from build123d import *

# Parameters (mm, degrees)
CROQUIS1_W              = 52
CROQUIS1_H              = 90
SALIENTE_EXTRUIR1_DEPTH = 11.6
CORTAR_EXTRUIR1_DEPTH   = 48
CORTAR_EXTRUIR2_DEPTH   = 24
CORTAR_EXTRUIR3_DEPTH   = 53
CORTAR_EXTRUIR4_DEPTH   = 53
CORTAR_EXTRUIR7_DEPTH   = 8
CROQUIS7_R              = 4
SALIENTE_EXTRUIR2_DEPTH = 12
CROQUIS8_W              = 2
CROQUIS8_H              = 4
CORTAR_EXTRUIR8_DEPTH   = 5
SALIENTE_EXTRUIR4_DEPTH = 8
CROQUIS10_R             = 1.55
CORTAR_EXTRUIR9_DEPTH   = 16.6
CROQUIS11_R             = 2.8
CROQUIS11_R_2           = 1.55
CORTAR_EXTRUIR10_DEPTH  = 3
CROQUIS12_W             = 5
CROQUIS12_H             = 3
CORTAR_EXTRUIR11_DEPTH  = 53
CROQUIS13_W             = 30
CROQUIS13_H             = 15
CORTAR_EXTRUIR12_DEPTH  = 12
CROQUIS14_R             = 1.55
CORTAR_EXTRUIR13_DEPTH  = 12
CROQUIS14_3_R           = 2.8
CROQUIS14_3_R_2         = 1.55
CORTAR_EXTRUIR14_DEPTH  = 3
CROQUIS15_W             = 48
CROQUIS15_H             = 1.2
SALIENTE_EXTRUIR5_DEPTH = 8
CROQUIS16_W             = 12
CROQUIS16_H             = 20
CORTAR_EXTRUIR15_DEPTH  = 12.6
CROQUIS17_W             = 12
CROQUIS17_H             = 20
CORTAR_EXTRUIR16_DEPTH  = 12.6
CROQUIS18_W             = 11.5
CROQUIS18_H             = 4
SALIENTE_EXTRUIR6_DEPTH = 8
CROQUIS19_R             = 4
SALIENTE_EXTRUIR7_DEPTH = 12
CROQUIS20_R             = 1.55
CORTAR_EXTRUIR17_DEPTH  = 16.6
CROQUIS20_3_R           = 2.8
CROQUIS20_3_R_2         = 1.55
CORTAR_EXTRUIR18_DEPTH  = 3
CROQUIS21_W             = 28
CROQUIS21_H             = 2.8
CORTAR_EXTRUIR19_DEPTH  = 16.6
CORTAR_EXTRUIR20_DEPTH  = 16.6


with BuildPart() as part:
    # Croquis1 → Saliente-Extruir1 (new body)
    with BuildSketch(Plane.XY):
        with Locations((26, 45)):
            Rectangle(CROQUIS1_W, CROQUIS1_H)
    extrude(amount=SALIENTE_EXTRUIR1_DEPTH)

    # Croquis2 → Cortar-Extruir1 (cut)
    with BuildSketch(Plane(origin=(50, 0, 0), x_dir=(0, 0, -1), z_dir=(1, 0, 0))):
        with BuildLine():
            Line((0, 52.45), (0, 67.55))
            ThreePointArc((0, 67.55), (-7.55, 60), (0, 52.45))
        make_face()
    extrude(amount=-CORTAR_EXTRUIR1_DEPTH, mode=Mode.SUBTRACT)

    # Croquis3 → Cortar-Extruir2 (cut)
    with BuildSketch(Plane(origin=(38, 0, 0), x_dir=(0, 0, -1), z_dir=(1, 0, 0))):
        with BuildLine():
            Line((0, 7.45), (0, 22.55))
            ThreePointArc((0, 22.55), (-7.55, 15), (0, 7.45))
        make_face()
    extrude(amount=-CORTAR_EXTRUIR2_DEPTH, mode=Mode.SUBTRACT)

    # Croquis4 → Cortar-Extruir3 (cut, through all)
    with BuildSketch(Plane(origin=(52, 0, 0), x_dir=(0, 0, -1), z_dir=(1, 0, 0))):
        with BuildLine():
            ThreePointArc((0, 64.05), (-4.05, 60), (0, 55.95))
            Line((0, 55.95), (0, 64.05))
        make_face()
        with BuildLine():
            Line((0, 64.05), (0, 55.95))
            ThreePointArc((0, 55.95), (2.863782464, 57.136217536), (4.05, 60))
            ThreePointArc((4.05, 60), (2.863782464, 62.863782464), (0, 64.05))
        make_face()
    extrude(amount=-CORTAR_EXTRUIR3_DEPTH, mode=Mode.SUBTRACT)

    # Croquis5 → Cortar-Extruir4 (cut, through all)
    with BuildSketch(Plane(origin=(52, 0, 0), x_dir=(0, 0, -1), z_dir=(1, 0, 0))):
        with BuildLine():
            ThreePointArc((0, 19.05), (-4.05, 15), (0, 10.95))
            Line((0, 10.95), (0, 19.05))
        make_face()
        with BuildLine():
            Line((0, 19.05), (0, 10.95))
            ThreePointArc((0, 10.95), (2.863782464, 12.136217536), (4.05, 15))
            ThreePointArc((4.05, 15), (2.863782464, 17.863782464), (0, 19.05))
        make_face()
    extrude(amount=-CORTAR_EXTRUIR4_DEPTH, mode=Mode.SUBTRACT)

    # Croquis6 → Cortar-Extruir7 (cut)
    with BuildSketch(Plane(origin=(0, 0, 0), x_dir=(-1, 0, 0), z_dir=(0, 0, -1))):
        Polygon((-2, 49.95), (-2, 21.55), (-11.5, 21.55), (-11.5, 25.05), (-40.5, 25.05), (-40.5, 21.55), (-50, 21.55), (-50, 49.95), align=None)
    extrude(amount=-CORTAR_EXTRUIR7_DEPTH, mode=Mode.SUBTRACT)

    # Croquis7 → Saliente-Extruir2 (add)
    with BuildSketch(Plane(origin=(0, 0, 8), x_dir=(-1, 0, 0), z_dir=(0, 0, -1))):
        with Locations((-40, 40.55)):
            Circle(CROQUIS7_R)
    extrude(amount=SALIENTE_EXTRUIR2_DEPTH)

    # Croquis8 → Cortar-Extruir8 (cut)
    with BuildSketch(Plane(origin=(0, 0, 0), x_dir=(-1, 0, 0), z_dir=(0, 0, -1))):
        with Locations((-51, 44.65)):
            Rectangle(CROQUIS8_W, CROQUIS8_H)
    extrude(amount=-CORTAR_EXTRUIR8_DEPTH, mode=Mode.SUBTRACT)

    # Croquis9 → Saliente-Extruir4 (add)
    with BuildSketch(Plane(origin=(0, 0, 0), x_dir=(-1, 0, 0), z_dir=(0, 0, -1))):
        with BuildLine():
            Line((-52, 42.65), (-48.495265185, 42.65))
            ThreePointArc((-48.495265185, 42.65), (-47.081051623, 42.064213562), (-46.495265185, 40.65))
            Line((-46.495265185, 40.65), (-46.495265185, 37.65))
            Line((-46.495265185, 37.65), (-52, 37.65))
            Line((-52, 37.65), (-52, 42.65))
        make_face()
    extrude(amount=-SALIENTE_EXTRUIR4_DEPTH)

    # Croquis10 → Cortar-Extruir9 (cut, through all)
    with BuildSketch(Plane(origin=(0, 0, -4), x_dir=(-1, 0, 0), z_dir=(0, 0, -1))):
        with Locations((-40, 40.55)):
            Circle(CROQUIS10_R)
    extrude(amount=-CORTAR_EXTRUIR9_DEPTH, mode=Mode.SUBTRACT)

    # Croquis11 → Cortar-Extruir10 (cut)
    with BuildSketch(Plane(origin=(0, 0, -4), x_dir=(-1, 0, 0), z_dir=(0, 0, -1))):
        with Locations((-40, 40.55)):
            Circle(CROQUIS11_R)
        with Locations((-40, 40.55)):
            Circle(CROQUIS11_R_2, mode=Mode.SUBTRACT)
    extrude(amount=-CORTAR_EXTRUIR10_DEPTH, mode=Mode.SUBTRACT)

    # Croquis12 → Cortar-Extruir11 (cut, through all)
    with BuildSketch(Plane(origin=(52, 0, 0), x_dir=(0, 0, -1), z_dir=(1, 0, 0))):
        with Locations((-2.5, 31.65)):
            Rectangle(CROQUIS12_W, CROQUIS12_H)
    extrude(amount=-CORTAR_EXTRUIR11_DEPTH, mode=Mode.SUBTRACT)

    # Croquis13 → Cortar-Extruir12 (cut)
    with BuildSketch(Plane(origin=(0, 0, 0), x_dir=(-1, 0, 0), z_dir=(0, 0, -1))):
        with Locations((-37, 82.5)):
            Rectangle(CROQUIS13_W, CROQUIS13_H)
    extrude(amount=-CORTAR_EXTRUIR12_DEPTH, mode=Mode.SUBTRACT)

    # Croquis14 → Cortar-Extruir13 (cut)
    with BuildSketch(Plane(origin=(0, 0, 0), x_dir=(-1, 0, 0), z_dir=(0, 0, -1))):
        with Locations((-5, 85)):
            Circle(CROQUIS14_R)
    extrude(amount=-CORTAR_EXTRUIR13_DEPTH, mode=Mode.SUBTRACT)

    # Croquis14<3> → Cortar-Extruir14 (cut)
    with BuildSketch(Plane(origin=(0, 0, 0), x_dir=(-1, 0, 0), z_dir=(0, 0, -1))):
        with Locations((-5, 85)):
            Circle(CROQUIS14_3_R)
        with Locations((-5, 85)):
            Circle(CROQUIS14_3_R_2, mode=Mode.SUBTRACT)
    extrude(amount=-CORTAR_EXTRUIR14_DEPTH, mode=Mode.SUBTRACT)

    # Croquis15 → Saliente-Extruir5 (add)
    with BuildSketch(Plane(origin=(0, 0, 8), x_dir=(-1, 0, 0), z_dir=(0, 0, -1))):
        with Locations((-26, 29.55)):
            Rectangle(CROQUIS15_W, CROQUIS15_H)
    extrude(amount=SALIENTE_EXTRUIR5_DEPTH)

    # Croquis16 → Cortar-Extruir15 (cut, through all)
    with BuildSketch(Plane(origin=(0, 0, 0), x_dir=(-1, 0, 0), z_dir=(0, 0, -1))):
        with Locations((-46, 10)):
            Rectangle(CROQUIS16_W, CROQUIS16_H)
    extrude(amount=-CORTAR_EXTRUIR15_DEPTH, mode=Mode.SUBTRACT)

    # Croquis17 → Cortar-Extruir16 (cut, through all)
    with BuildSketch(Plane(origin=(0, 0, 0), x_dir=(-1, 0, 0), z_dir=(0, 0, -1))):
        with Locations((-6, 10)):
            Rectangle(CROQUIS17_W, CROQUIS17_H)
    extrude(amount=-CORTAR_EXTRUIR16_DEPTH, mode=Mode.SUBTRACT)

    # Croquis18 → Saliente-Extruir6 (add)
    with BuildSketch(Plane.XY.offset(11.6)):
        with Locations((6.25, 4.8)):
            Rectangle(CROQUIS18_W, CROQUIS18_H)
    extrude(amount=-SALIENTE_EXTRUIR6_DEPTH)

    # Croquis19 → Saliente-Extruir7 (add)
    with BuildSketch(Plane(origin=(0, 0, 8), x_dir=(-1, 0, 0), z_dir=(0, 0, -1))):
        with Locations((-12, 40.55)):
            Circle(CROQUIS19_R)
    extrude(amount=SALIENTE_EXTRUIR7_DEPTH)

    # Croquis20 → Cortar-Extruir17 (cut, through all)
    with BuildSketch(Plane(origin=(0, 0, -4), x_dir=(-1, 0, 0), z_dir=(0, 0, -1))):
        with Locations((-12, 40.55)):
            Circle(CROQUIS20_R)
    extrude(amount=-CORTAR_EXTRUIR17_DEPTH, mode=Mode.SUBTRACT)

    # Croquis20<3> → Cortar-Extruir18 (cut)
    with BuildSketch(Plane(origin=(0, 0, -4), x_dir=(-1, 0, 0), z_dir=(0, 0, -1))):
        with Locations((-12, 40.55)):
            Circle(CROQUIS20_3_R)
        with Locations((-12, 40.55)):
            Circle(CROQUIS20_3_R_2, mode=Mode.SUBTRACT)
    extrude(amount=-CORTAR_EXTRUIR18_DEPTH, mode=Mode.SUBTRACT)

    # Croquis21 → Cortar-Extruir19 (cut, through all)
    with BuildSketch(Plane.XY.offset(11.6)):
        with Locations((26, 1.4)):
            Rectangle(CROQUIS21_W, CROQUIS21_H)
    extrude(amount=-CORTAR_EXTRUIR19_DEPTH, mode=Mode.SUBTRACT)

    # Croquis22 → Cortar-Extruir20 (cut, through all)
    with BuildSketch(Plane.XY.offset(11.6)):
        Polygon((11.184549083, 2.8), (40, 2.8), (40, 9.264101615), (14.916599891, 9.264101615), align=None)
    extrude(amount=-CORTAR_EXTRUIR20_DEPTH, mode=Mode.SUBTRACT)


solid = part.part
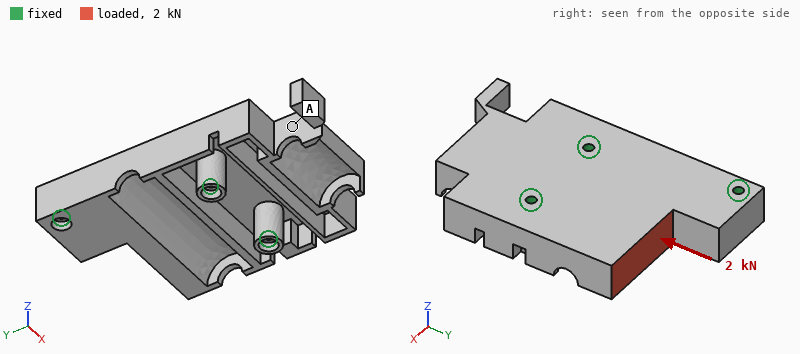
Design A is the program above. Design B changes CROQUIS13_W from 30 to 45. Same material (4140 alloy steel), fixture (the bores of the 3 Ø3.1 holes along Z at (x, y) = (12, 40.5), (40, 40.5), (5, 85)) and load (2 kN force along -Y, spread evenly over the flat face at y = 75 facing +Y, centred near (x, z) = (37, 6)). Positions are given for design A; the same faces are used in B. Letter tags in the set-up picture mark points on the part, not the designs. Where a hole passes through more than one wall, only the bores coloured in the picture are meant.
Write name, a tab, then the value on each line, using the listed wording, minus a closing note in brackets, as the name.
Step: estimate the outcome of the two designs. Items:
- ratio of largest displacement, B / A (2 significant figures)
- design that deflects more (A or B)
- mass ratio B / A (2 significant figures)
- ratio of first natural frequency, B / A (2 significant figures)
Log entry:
ratio of largest displacement, B / A	1.1
design that deflects more	B
mass ratio B / A	0.95
ratio of first natural frequency, B / A	1.00
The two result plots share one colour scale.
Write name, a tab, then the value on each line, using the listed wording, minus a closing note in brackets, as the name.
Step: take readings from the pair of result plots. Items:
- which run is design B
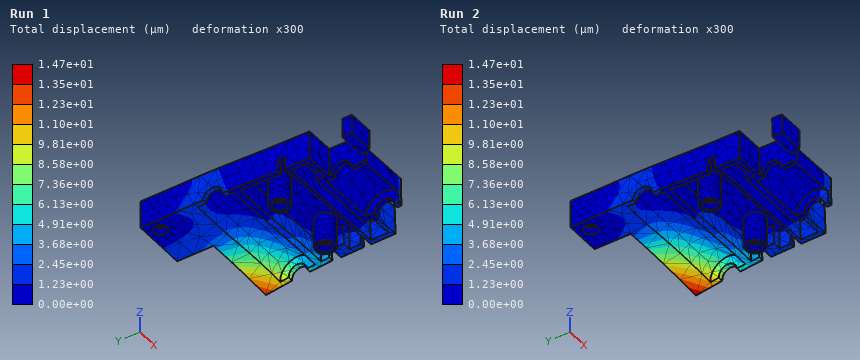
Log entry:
which run is design B	Run 2
